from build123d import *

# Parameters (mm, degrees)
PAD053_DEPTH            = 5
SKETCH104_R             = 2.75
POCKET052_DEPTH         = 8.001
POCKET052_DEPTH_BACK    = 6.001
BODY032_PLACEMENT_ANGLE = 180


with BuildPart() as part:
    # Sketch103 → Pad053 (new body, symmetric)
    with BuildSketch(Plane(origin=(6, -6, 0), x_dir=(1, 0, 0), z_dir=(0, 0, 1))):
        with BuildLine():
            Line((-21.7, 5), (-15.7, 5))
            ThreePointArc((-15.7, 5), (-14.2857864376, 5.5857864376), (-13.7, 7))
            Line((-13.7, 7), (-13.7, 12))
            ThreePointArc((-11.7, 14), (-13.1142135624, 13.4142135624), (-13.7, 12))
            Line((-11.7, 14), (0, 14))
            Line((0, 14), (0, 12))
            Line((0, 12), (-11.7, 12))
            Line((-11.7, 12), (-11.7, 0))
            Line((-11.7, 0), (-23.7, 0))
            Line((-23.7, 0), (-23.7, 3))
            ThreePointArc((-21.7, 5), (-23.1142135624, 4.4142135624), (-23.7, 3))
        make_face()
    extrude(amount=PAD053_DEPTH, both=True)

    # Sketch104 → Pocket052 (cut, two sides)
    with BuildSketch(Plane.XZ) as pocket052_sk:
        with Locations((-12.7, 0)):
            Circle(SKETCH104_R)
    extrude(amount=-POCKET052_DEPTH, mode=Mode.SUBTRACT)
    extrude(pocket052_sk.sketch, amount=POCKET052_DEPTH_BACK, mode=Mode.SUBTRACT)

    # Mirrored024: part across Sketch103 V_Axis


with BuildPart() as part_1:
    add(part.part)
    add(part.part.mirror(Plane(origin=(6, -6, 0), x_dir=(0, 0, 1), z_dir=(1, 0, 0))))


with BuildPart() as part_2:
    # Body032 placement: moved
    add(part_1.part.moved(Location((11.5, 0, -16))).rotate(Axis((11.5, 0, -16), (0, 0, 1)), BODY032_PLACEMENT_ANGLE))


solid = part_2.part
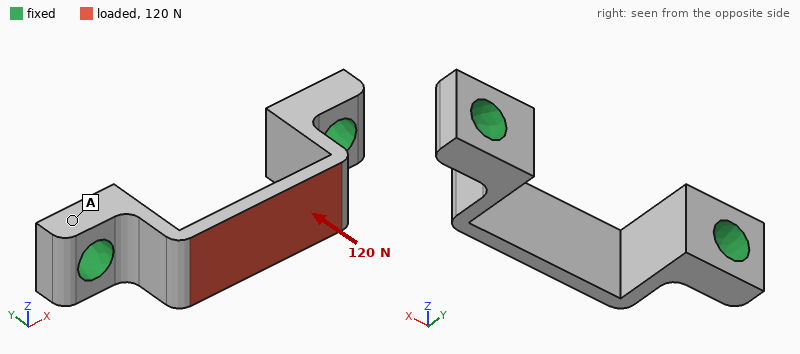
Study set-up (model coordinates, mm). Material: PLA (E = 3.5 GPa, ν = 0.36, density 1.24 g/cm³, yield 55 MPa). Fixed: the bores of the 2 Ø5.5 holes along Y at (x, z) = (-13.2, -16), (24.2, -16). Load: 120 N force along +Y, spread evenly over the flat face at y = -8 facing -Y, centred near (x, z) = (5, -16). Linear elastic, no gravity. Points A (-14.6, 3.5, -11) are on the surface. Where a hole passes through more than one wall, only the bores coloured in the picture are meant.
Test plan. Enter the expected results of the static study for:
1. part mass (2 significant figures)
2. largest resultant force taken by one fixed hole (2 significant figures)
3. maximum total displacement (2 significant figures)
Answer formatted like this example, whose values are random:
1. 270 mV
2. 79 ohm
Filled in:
1. 2.2 g
2. 75 N
3. 0.36 mm
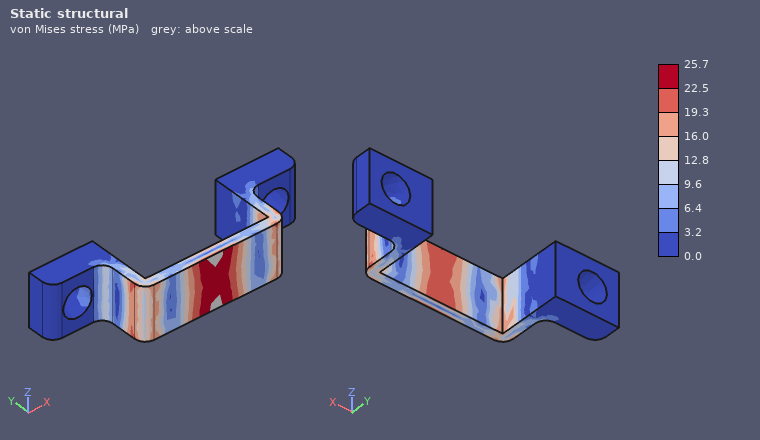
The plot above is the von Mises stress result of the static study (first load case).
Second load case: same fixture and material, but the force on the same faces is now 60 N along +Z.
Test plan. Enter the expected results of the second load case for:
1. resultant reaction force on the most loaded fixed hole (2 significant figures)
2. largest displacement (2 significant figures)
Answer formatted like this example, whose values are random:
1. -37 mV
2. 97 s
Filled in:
1. 30 N
2. 100 µm
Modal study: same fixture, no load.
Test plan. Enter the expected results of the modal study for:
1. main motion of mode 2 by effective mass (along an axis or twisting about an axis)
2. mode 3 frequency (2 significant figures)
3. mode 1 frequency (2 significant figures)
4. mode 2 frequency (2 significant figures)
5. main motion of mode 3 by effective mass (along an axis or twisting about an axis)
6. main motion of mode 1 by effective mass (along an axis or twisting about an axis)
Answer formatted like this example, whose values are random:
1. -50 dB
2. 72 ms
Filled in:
1. along Y
2. 5500 Hz
3. 4000 Hz
4. 4400 Hz
5. along Z
6. along X
